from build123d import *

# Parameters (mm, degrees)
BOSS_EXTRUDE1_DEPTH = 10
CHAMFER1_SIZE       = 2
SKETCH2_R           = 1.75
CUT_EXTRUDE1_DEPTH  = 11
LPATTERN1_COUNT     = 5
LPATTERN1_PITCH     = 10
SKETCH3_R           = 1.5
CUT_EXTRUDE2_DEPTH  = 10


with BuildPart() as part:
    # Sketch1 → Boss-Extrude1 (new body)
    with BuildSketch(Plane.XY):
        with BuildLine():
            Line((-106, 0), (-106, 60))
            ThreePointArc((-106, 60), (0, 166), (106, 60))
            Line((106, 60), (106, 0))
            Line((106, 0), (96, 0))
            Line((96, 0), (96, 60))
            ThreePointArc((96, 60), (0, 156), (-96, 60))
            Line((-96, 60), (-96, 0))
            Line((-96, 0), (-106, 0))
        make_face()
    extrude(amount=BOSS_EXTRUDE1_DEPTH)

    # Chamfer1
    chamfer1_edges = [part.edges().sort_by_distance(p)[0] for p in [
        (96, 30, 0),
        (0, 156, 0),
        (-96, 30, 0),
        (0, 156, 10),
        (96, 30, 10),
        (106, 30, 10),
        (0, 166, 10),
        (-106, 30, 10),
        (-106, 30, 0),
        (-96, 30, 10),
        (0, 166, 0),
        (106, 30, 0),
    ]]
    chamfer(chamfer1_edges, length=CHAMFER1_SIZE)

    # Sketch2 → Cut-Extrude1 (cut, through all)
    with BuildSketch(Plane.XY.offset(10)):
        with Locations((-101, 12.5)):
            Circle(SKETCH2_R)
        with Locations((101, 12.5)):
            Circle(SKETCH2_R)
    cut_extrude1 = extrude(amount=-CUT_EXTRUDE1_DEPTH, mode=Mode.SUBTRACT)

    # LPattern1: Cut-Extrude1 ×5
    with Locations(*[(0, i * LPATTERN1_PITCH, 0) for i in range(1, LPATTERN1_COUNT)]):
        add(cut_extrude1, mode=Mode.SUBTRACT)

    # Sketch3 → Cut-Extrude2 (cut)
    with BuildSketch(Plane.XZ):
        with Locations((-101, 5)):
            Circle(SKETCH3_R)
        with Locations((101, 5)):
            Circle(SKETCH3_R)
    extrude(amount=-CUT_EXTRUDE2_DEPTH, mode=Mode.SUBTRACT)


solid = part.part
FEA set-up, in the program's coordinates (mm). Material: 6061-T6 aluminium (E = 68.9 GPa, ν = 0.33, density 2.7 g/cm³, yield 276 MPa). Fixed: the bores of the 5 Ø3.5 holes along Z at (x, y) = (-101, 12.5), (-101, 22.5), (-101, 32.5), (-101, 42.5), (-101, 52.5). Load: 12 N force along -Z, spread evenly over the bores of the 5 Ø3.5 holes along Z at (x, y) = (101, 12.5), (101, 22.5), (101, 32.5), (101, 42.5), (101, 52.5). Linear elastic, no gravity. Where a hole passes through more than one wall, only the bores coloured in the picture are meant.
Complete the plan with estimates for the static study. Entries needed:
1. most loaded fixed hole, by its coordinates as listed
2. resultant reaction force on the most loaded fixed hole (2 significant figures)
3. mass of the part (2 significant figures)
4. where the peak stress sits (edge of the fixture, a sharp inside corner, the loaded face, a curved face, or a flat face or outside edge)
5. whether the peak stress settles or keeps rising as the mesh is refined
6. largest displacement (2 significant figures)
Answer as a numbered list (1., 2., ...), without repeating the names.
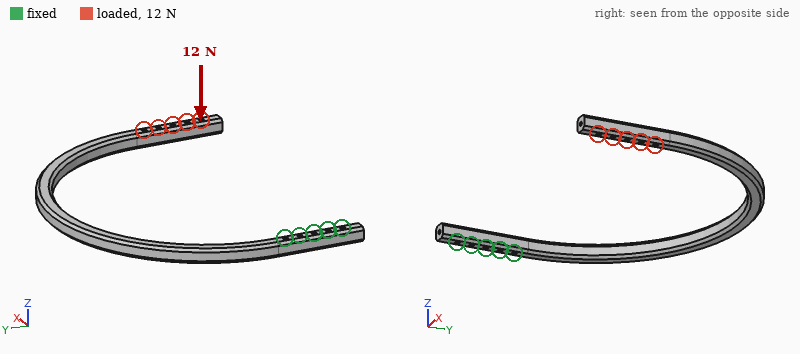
1. (-101, 52.5)
2. 9.9 N
3. 110 g
4. edge of the fixture
5. keeps rising
6. 3.1 mm
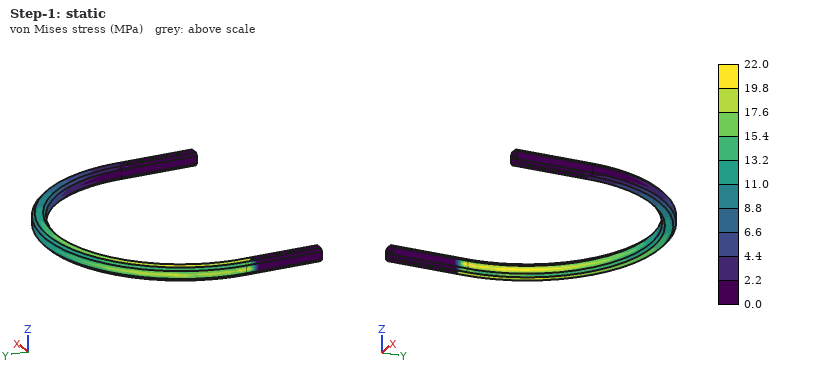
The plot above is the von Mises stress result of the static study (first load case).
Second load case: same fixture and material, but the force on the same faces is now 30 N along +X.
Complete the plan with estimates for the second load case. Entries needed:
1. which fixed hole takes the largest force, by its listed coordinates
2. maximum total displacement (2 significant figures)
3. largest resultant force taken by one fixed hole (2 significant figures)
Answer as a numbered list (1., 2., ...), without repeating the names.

1. (-101, 42.5)
2. 3.2 mm
3. 23 N
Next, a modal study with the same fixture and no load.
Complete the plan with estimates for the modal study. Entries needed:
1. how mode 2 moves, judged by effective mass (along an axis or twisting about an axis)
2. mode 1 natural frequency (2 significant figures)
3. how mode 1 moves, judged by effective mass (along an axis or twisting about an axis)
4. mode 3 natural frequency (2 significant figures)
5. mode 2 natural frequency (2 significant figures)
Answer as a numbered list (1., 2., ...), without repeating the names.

1. along Y
2. 62 Hz
3. along Z
4. 180 Hz
5. 70 Hz
